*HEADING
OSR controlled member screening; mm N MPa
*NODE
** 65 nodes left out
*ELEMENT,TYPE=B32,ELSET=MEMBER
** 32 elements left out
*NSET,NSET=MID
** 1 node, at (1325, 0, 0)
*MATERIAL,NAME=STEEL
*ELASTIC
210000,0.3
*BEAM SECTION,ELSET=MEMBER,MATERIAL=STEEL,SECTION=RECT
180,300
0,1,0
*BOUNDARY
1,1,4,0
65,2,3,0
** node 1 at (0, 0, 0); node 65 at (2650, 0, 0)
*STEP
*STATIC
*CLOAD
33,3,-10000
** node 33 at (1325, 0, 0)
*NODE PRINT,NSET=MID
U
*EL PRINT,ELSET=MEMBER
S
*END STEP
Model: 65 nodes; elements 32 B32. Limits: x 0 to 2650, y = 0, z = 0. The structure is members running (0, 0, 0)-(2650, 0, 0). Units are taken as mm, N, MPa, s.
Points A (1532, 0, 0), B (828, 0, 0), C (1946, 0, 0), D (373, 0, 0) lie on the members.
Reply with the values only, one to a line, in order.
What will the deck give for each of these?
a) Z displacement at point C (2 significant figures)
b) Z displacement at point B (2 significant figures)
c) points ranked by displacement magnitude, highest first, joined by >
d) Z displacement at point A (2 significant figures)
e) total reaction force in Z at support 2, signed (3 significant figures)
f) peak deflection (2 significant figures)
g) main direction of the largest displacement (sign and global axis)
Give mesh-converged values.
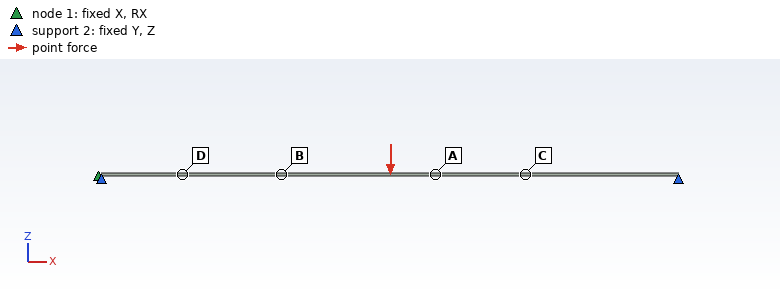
-0.034 mm
-0.038 mm
A > B > C > D
-0.046 mm
10000 N
0.047 mm
-Z
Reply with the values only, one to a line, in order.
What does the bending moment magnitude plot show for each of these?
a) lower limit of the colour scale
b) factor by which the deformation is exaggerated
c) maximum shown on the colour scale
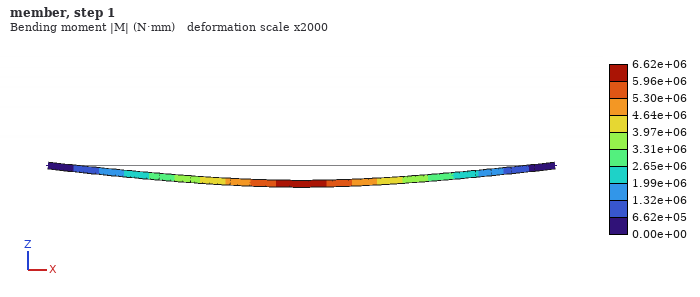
0.00e+00 N·mm
2000
6.62e+06 N·mm
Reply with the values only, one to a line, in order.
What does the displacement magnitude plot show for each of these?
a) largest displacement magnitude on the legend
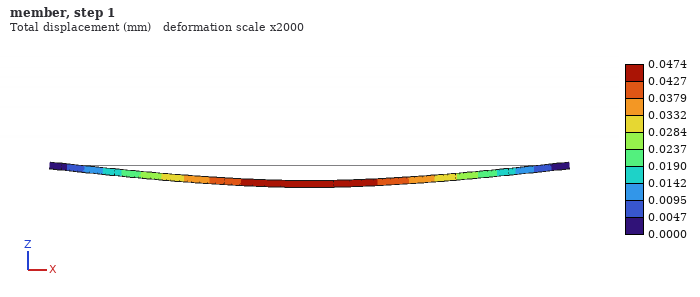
0.0474 mm
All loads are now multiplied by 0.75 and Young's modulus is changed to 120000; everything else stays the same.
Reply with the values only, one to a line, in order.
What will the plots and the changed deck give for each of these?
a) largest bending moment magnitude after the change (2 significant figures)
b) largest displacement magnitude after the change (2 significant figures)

5.0e+06 N·mm
0.062 mm
